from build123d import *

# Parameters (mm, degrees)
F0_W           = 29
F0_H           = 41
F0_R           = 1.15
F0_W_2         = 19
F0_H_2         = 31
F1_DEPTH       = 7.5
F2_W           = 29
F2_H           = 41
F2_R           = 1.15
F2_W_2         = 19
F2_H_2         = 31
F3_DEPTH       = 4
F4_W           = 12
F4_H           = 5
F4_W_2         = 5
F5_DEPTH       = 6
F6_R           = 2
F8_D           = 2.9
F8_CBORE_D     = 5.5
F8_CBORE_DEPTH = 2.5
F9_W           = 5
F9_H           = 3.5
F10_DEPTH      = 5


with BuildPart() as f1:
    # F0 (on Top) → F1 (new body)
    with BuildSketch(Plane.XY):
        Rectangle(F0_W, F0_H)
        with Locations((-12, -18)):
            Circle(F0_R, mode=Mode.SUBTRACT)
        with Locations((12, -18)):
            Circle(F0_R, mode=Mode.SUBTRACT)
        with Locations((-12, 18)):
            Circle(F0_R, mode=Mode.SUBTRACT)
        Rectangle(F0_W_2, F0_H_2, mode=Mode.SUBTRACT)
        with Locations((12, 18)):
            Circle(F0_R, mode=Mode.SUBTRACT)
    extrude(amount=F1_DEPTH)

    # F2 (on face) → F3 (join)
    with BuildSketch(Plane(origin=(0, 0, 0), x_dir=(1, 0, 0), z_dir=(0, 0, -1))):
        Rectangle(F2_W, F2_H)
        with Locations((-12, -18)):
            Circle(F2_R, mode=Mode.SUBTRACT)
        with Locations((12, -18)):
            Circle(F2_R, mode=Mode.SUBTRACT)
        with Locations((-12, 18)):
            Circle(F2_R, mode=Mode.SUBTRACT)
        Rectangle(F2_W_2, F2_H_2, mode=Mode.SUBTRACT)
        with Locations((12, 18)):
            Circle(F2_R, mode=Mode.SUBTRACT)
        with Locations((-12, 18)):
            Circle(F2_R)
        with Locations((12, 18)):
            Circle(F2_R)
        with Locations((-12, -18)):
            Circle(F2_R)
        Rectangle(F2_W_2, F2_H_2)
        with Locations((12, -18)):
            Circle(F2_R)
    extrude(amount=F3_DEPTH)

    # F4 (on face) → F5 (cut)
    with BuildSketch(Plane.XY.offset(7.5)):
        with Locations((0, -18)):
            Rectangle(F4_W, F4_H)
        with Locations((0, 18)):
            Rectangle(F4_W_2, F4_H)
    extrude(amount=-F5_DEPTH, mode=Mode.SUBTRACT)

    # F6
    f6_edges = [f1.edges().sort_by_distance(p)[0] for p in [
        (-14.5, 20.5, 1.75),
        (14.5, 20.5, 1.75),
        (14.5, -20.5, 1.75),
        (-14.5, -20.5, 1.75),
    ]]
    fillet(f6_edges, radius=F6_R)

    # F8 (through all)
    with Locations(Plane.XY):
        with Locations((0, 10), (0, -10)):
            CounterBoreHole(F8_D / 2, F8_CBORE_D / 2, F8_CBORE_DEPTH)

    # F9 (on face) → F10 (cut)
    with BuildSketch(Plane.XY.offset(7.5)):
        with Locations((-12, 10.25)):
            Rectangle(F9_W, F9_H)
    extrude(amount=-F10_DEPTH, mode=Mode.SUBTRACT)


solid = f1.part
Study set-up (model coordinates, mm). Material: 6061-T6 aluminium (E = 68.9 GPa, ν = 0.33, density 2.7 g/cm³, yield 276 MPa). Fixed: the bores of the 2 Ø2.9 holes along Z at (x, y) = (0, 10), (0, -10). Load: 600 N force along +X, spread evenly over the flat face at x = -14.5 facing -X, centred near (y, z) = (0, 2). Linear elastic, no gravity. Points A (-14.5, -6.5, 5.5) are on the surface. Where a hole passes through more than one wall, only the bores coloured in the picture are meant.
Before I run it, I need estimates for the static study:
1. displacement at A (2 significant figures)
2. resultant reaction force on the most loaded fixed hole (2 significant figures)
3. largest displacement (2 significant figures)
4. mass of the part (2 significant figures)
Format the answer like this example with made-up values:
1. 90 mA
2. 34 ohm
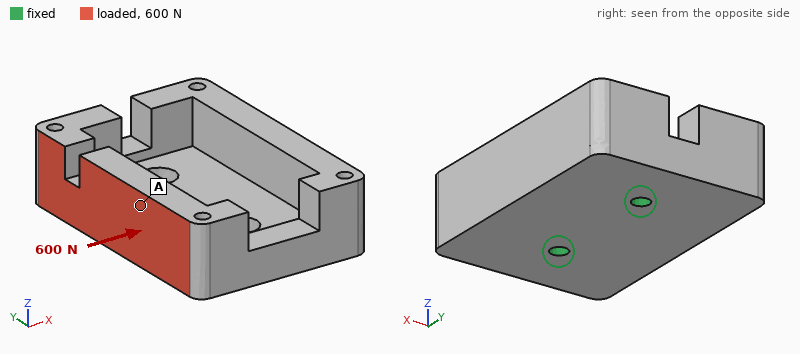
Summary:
1. 68 µm
2. 320 N
3. 73 µm
4. 23 g
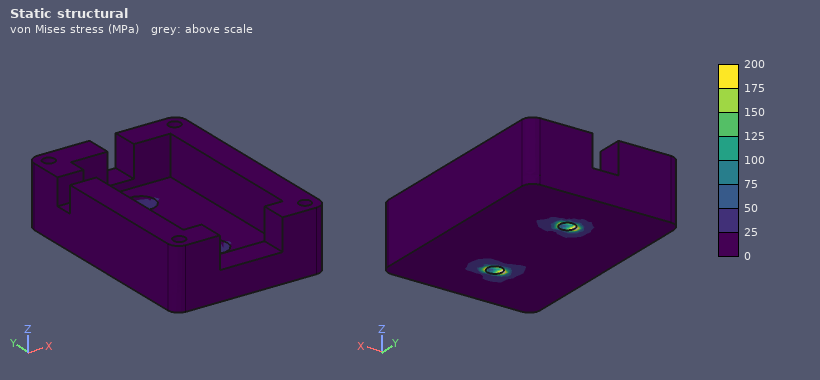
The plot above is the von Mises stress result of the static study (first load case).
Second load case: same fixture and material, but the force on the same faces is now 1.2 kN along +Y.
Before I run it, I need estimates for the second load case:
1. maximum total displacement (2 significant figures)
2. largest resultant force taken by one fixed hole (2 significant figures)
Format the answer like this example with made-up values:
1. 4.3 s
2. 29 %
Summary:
1. 25 µm
2. 1.1 kN
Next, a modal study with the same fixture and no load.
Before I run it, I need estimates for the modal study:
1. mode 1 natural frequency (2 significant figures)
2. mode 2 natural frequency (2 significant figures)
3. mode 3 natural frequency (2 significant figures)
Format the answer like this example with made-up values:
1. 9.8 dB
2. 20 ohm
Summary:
1. 2900 Hz
2. 8700 Hz
3. 8900 Hz
